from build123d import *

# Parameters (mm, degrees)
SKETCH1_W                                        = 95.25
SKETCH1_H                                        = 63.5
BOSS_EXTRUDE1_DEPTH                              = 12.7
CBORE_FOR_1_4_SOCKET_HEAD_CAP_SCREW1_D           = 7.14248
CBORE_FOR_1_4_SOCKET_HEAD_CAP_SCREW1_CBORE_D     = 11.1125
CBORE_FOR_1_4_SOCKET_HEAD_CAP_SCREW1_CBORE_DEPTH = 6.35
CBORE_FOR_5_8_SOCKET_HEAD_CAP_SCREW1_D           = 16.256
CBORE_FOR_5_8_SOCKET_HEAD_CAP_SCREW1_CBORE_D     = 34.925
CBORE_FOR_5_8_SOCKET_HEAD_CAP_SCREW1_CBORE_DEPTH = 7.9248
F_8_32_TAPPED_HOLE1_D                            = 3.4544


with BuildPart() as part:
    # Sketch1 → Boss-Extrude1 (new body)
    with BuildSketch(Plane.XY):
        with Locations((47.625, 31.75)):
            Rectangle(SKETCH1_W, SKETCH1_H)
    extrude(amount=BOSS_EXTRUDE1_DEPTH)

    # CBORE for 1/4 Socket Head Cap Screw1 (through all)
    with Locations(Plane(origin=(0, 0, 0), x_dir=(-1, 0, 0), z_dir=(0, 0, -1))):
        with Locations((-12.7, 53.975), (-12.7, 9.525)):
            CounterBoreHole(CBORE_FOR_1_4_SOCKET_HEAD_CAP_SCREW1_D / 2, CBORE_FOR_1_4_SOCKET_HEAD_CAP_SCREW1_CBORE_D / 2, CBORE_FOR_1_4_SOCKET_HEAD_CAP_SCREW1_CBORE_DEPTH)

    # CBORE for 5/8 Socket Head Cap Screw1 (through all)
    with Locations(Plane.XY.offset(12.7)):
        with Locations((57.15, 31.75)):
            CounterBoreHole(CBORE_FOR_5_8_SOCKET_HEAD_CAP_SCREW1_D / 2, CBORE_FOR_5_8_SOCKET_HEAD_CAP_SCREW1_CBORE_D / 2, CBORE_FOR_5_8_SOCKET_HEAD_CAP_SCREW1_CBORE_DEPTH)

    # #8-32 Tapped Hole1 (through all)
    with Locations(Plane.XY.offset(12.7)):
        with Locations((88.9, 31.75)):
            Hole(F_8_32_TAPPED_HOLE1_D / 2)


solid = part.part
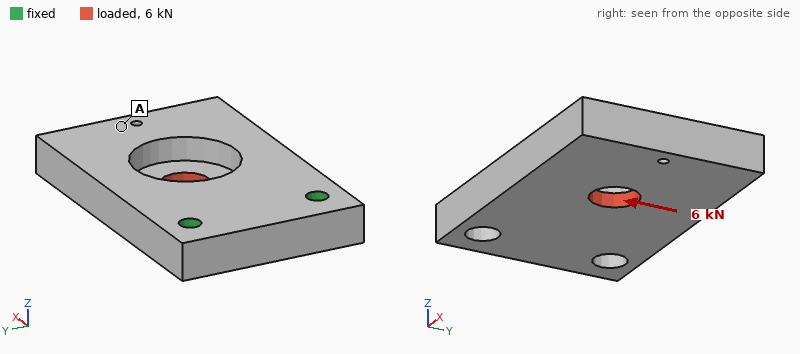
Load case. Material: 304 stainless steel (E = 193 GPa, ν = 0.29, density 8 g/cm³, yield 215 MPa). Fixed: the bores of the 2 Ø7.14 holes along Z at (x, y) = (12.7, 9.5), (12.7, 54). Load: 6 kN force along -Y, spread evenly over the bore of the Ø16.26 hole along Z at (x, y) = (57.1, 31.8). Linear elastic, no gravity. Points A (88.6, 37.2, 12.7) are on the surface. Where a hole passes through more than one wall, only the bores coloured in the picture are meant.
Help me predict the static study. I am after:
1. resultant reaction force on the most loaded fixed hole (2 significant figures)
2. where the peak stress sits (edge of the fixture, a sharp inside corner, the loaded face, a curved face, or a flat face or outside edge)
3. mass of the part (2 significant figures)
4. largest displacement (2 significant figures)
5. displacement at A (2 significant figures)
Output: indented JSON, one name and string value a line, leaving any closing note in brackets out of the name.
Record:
{
  "resultant reaction force on the most loaded fixed hole": "6.4 kN",
  "where the peak stress sits": "edge of the fixture",
  "mass of the part": "530 g",
  "largest displacement": "22 µm",
  "displacement at A": "19 µm"
}
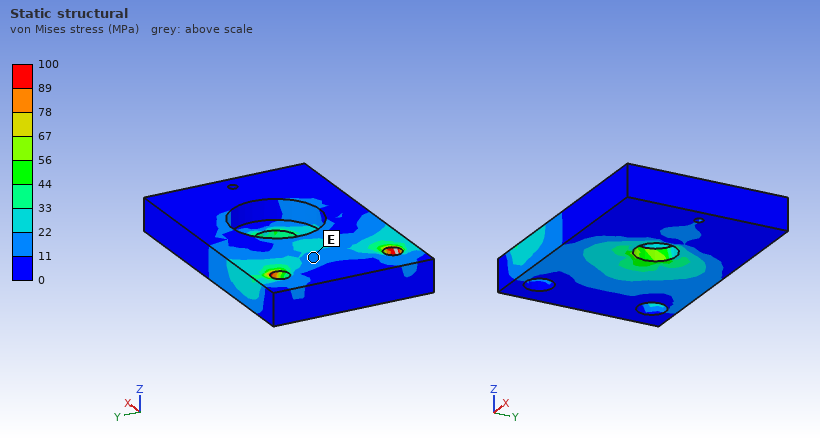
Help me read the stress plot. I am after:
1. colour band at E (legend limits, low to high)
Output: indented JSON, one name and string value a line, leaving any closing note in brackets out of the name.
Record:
{
  "colour band at E": "11 to 22 MPa"
}
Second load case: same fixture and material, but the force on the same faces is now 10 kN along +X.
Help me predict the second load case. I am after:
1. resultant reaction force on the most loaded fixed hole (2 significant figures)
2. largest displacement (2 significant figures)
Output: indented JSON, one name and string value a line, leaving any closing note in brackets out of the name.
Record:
{
  "resultant reaction force on the most loaded fixed hole": "5.0 kN",
  "largest displacement": "0.11 mm"
}
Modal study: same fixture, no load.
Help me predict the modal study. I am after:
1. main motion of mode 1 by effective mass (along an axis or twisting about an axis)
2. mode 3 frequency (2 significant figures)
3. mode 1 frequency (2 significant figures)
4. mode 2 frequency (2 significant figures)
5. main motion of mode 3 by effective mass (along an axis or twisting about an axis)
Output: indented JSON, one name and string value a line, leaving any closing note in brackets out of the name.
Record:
{
  "main motion of mode 1 by effective mass": "along Z",
  "mode 3 frequency": "4700 Hz",
  "mode 1 frequency": "1100 Hz",
  "mode 2 frequency": "3200 Hz",
  "main motion of mode 3 by effective mass": "along Y"
}
